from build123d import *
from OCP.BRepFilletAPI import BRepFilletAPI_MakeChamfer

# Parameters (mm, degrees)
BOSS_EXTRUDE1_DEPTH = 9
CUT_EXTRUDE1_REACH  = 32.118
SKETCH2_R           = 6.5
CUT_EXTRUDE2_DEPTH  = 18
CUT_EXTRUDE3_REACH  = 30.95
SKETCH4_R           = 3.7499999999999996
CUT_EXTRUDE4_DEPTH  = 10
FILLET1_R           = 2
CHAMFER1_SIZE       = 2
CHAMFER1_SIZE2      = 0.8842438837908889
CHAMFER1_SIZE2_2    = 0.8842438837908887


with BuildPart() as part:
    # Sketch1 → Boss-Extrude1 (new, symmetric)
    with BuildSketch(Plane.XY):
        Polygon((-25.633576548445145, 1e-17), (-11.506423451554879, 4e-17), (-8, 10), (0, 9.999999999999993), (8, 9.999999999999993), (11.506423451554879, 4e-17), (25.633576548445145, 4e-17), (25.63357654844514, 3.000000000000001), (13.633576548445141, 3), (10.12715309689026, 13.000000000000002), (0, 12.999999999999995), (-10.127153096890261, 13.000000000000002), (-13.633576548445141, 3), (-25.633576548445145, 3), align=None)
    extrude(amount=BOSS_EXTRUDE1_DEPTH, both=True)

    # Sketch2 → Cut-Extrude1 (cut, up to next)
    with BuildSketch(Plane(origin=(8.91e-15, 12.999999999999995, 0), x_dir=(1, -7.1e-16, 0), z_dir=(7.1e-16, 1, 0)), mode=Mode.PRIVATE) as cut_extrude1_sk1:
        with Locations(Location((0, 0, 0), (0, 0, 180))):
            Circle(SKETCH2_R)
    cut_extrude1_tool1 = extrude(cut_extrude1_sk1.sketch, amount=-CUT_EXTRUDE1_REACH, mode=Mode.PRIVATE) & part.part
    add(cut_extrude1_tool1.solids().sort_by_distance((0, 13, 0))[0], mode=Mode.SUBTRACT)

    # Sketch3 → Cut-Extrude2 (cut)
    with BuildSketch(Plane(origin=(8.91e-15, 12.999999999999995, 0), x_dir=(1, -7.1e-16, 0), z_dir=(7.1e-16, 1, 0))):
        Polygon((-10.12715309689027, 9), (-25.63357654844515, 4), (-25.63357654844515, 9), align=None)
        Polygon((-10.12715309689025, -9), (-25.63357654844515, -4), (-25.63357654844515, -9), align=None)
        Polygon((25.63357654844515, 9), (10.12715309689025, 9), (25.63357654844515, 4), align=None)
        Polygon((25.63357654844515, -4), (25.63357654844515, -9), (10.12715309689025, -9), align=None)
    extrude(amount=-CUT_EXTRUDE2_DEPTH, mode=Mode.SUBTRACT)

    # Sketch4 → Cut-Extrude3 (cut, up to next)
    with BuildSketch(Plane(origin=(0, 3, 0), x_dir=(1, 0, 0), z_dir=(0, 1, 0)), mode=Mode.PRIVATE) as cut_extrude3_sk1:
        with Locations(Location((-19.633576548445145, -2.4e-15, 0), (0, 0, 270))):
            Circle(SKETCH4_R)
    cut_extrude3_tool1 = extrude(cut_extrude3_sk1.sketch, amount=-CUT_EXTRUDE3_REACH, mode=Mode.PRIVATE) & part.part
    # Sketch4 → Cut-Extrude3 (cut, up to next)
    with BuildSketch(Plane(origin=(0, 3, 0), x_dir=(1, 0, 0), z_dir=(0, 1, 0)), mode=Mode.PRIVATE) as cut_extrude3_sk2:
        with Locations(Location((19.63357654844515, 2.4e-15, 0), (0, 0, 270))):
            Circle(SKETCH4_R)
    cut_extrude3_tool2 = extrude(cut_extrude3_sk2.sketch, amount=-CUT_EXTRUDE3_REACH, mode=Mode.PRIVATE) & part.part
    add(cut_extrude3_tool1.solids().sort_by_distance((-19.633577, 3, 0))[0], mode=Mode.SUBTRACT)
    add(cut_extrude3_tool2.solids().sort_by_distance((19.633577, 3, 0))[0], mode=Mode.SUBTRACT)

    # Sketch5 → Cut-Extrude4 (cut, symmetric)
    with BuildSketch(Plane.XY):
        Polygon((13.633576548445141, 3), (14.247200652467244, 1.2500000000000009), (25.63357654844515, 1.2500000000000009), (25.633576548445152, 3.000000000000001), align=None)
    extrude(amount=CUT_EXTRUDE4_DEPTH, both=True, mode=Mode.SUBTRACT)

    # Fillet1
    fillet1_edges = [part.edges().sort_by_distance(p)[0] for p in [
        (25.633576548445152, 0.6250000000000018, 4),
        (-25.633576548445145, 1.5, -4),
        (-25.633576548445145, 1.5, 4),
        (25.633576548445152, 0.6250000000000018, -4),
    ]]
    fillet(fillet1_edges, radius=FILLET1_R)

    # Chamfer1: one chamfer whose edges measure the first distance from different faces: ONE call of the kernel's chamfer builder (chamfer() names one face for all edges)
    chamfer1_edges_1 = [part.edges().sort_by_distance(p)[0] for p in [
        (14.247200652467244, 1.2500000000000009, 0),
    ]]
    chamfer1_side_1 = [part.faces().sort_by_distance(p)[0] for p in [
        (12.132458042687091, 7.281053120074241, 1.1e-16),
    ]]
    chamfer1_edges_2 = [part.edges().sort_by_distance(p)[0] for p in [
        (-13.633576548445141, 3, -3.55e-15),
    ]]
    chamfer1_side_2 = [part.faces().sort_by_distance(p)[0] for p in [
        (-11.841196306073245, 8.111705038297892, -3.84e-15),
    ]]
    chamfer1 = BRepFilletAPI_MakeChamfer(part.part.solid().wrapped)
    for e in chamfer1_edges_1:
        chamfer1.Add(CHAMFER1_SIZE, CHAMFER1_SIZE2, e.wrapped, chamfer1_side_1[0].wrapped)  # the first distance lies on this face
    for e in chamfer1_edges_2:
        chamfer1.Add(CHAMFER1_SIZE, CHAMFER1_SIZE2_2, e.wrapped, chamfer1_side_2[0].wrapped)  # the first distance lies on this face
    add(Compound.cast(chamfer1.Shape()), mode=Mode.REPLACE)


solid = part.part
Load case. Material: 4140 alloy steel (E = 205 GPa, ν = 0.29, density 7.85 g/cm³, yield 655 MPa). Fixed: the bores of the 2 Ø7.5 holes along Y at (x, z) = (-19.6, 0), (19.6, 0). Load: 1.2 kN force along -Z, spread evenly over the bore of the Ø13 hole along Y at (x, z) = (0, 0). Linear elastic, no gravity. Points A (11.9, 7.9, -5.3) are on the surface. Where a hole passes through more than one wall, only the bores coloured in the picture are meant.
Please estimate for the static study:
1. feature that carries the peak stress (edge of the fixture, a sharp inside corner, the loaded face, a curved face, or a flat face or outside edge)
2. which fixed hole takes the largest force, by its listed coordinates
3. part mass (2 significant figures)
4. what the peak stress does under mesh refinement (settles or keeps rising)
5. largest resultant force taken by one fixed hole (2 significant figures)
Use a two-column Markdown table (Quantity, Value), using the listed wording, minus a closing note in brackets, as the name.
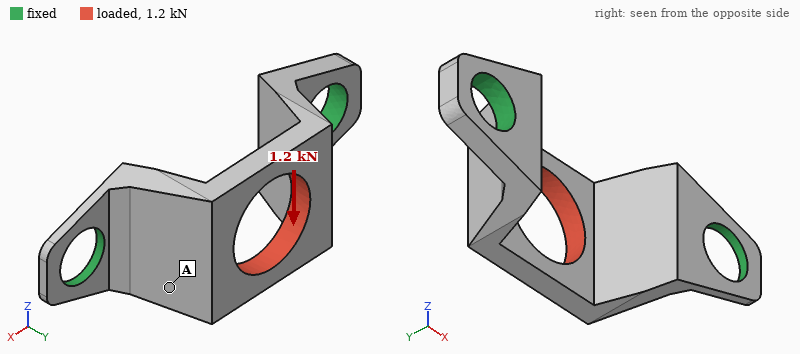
| Quantity | Value |
|---|---|
| feature that carries the peak stress | edge of the fixture |
| which fixed hole takes the largest force, by its listed coordinates | (-19.6, 0) |
| part mass | 18 g |
| what the peak stress does under mesh refinement | keeps rising |
| largest resultant force taken by one fixed hole | 770 N |
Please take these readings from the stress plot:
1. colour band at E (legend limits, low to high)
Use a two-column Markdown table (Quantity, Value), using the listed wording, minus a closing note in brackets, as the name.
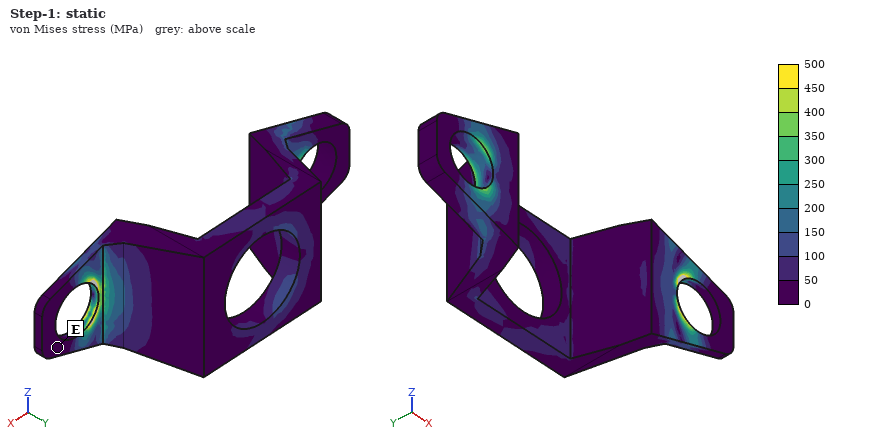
| Quantity | Value |
|---|---|
| colour band at E | 0 to 50 MPa |
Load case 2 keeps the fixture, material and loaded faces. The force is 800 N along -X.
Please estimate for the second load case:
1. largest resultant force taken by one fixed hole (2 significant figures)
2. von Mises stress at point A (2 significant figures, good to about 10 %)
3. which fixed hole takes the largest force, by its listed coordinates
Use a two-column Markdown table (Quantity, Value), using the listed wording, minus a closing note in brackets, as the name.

| Quantity | Value |
|---|---|
| largest resultant force taken by one fixed hole | 530 N |
| von Mises stress at point A | 25 MPa |
| which fixed hole takes the largest force, by its listed coordinates | (-19.6, 0) |
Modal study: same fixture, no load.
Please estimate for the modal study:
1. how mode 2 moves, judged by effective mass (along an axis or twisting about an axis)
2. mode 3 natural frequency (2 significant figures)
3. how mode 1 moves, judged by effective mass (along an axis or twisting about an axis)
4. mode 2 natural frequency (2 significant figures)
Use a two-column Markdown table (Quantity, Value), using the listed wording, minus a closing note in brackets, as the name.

| Quantity | Value |
|---|---|
| how mode 2 moves, judged by effective mass | along X |
| mode 3 natural frequency | 15 kHz |
| how mode 1 moves, judged by effective mass | along Z |
| mode 2 natural frequency | 12 kHz |
